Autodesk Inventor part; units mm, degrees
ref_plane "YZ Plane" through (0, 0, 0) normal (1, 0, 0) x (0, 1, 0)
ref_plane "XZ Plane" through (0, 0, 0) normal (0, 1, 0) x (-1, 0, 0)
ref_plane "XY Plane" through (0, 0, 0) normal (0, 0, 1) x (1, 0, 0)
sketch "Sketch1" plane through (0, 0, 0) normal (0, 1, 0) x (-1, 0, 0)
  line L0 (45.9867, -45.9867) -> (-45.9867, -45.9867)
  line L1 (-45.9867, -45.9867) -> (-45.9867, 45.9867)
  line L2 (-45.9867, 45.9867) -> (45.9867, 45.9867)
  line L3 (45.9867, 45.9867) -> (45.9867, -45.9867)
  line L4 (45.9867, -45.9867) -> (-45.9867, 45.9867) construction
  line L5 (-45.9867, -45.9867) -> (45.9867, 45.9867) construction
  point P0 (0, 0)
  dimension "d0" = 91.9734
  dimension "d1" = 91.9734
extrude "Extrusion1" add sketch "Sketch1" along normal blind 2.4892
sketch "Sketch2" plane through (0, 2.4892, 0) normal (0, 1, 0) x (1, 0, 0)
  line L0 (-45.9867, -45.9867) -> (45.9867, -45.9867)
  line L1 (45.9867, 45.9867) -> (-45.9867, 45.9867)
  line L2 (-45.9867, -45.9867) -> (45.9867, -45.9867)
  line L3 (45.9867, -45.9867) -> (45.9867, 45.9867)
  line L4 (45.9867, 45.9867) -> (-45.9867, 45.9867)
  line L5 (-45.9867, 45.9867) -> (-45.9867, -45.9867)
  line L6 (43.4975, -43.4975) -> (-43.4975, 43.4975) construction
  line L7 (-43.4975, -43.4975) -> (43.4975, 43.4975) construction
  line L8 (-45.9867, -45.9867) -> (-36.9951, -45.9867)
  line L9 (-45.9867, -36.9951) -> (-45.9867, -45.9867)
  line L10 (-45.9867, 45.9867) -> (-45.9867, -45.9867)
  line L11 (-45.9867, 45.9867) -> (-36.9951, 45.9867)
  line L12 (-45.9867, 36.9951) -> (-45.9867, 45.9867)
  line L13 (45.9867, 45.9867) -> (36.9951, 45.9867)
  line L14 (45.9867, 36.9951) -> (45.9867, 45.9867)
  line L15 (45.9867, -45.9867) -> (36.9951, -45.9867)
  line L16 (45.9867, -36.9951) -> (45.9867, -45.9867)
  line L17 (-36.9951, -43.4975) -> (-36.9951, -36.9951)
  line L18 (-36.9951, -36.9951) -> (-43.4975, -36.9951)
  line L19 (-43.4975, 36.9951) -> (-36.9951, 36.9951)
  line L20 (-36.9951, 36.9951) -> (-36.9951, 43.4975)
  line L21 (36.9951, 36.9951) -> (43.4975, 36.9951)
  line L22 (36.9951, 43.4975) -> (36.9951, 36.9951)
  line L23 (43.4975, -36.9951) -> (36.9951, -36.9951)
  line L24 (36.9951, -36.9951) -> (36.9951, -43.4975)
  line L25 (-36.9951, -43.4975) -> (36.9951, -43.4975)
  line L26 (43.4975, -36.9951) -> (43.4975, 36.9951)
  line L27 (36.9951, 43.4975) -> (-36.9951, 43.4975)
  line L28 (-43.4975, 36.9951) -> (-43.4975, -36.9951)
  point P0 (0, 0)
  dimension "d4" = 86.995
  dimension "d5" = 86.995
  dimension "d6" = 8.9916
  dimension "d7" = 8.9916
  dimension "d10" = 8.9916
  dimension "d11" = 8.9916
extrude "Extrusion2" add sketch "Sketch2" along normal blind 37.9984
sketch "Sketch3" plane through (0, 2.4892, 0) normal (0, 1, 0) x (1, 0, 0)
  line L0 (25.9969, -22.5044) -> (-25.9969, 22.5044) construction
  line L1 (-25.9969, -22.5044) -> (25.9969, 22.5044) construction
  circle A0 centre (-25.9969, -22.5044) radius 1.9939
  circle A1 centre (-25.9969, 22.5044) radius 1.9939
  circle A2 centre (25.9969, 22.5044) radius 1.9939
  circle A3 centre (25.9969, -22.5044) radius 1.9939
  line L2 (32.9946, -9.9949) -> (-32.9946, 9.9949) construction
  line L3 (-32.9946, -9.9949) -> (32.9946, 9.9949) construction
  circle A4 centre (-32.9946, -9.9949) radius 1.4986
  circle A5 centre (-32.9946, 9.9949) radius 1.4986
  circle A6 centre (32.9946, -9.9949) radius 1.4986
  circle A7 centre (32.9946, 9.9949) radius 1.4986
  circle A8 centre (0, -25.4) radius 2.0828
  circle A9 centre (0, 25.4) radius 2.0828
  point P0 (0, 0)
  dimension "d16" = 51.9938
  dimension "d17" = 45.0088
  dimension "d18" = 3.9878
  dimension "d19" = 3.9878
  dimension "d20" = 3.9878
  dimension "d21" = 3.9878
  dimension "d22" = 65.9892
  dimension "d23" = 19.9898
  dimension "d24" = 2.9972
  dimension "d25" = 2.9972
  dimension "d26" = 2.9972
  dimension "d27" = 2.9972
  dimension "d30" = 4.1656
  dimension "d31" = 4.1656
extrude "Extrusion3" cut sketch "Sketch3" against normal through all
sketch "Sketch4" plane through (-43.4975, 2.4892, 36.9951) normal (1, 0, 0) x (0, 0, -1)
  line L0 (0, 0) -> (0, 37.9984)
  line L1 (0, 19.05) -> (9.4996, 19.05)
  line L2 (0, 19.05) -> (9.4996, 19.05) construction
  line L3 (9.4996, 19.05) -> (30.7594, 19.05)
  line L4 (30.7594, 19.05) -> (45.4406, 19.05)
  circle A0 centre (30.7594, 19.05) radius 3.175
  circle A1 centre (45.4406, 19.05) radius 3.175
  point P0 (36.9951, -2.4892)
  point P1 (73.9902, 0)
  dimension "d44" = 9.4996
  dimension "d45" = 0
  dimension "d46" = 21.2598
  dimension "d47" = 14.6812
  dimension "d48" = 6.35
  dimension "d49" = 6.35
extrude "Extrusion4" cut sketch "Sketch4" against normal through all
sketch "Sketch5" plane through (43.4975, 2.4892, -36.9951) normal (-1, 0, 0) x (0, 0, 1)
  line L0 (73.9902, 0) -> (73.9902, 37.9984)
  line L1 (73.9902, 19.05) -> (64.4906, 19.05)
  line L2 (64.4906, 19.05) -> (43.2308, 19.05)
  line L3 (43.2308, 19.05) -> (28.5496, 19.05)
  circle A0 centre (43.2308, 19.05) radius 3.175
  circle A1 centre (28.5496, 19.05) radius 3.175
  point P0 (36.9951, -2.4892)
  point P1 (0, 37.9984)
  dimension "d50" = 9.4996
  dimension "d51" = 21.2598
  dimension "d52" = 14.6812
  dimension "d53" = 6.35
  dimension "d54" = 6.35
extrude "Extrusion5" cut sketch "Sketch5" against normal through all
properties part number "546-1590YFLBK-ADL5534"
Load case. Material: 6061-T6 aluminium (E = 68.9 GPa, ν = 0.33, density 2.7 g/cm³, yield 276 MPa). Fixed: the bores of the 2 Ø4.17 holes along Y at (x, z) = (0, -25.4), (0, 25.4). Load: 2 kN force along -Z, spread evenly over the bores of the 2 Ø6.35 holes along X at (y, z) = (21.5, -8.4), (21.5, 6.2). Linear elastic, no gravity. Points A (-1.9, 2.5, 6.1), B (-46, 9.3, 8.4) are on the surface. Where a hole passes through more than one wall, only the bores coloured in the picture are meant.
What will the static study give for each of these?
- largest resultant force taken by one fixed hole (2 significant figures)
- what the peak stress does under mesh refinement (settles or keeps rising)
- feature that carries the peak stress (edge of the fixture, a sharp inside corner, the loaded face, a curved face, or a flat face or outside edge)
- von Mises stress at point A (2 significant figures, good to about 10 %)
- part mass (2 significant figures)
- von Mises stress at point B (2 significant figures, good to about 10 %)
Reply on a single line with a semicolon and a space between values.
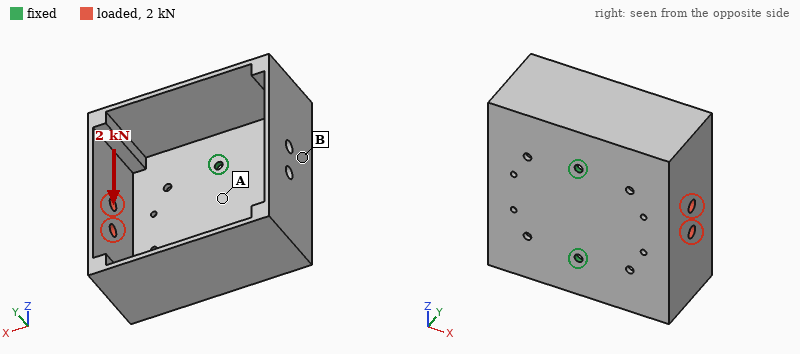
2.1 kN; keeps rising; edge of the fixture; 19 MPa; 160 g; 54 MPa
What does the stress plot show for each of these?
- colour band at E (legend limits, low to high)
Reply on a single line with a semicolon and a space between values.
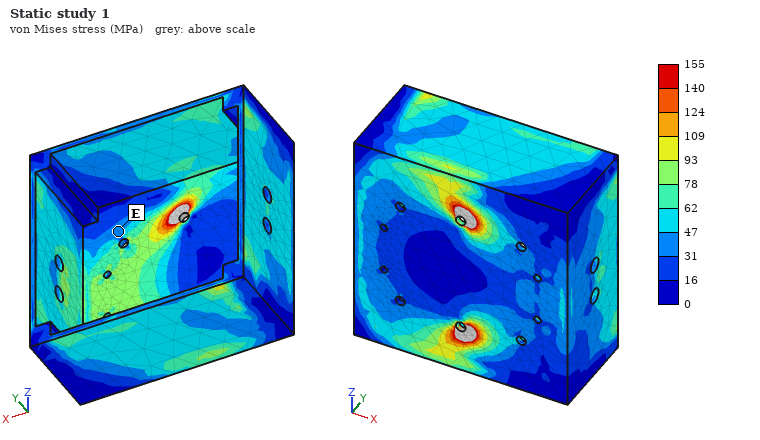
31 to 47 MPa
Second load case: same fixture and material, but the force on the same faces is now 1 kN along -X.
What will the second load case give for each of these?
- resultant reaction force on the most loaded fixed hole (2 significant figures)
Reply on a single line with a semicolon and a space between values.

550 N
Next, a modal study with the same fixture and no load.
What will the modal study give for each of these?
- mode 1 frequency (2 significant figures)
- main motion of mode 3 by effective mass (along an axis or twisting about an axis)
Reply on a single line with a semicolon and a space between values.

340 Hz; along Z
